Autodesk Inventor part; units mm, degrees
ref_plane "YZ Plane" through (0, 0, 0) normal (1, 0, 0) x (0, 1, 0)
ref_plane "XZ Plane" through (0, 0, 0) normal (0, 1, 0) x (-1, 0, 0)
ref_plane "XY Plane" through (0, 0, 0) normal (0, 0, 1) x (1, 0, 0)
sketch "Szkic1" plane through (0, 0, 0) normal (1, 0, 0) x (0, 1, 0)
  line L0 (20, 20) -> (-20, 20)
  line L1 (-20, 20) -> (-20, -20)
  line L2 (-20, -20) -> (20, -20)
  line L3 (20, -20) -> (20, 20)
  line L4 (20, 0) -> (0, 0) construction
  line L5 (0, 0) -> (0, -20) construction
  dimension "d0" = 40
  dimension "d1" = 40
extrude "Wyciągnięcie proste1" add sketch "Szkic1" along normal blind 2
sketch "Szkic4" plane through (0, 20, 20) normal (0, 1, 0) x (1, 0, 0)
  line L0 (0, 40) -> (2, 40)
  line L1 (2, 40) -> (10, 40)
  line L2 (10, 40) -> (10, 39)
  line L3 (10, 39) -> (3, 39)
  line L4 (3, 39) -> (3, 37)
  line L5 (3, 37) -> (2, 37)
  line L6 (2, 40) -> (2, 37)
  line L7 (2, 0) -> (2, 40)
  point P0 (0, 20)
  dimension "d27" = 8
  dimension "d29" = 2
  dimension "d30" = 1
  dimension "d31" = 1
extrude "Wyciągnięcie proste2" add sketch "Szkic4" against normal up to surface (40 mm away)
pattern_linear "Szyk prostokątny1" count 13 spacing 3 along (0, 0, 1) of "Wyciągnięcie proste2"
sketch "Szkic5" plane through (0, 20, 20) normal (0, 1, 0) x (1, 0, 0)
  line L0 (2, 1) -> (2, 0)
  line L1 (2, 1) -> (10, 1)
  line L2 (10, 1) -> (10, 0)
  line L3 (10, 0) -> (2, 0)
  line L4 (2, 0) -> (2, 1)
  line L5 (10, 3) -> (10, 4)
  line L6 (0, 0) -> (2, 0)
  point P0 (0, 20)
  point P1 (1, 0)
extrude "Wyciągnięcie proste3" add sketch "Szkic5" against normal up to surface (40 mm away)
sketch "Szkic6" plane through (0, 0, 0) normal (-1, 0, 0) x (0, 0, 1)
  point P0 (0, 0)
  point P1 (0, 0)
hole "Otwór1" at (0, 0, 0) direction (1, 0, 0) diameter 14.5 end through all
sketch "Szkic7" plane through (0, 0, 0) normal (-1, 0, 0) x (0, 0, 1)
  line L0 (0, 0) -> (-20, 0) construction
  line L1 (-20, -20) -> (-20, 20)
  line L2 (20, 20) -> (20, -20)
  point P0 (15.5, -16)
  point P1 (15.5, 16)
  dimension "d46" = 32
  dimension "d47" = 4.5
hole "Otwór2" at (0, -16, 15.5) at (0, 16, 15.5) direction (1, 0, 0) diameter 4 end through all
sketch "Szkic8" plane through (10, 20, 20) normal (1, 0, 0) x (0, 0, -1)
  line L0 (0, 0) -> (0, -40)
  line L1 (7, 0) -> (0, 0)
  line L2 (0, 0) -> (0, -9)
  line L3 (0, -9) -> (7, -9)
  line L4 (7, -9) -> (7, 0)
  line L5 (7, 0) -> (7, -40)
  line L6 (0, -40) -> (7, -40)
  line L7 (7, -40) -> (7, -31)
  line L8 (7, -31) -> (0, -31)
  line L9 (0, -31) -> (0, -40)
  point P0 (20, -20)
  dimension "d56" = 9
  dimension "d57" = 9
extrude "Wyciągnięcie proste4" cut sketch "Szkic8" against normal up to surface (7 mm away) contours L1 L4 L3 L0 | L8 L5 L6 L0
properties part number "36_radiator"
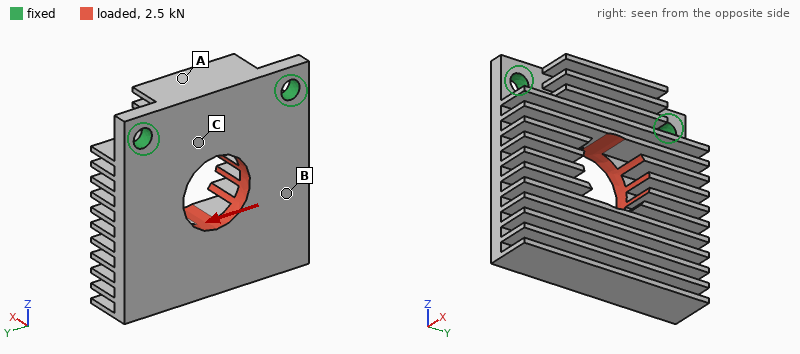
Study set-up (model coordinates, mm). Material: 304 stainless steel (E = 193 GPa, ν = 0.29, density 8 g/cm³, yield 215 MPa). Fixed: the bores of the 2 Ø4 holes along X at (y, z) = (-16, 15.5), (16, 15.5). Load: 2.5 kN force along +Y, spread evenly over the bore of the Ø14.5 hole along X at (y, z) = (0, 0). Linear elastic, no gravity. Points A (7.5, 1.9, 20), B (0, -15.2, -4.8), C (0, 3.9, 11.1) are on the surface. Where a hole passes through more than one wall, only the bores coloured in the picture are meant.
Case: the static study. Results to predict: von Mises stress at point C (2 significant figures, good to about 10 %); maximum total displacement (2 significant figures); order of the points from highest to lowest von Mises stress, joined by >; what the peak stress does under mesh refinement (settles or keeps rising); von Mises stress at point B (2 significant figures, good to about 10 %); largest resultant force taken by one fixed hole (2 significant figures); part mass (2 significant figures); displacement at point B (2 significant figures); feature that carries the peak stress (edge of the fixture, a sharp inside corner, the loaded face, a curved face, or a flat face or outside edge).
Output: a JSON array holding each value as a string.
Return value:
["34 MPa", "45 µm", "C > B > A", "keeps rising", "21 MPa", "1.7 kN", "59 g", "20 µm", "edge of the fixture"]
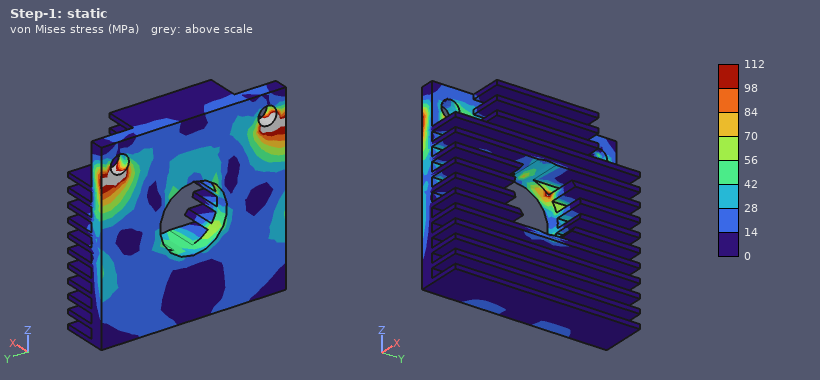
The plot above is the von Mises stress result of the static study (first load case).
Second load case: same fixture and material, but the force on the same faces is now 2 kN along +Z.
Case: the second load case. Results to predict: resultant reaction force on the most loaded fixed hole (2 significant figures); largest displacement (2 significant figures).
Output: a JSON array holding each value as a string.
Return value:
["1.0 kN", "0.13 mm"]
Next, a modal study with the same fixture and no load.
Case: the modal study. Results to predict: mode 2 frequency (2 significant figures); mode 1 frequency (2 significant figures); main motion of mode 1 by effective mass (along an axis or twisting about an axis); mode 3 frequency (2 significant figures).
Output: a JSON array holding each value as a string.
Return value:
["3000 Hz", "1300 Hz", "along X", "7000 Hz"]
